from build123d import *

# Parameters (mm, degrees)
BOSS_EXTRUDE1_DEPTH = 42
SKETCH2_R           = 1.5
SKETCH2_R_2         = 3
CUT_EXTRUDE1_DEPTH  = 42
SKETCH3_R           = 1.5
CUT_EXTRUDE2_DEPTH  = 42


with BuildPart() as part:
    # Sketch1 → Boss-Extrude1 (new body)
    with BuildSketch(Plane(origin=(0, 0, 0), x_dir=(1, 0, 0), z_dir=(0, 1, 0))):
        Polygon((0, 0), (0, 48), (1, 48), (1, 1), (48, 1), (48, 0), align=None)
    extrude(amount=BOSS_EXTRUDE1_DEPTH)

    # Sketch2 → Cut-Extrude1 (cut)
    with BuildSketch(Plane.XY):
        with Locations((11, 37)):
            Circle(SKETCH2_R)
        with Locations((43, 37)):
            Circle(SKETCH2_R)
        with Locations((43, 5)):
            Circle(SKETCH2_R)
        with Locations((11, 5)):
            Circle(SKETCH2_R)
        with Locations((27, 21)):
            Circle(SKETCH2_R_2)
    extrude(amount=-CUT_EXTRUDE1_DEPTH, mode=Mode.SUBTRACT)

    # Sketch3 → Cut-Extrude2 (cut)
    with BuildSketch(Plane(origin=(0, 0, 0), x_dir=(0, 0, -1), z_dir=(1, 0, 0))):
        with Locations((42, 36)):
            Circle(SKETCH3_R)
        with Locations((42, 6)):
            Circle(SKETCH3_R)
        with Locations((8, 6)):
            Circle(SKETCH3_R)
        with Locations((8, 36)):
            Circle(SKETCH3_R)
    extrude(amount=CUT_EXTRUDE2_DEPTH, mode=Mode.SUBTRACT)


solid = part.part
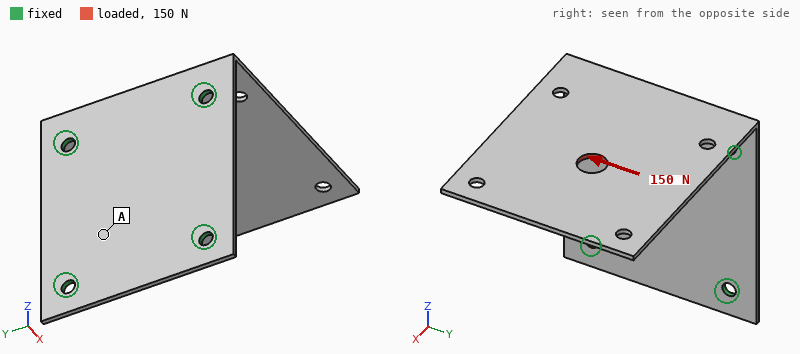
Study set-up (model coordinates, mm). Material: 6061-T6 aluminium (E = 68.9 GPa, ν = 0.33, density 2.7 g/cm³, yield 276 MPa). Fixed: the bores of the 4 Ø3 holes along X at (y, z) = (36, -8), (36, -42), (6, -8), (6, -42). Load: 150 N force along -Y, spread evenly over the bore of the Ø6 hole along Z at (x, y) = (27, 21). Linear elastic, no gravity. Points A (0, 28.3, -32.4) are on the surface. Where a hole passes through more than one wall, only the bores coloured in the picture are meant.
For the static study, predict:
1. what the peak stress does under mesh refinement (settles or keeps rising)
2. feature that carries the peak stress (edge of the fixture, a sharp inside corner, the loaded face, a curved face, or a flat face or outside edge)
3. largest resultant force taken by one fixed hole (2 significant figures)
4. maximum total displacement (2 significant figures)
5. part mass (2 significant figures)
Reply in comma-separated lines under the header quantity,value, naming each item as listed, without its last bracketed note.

quantity,value
what the peak stress does under mesh refinement,keeps rising
feature that carries the peak stress,edge of the fixture
largest resultant force taken by one fixed hole,150 N
maximum total displacement,0.52 mm
part mass,11 g
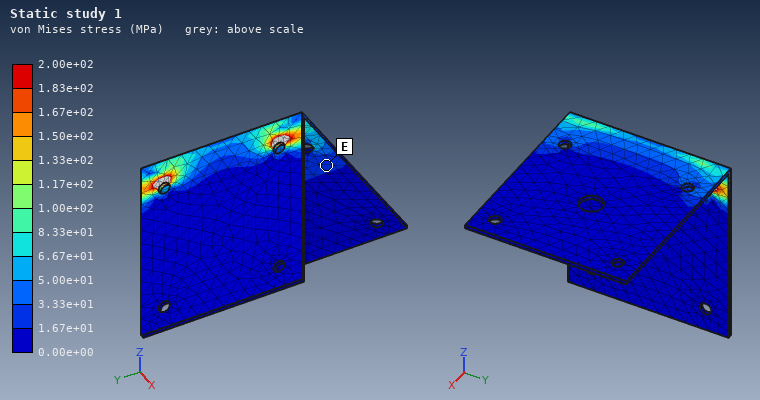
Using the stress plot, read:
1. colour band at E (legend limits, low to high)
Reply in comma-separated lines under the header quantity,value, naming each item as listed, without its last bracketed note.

quantity,value
colour band at E,1.67e+01 to 3.33e+01 MPa
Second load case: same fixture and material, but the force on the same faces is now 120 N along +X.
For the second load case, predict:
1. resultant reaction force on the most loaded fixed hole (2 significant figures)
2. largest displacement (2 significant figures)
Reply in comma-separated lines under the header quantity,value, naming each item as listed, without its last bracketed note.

quantity,value
resultant reaction force on the most loaded fixed hole,62 N
largest displacement,0.63 mm
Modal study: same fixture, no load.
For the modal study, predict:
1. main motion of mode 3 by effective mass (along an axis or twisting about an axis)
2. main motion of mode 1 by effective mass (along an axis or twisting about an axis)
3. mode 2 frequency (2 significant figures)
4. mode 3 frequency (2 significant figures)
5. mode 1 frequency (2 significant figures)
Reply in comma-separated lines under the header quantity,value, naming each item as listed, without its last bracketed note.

quantity,value
main motion of mode 3 by effective mass,along Y
main motion of mode 1 by effective mass,along Z
mode 2 frequency,890 Hz
mode 3 frequency,1700 Hz
mode 1 frequency,300 Hz
